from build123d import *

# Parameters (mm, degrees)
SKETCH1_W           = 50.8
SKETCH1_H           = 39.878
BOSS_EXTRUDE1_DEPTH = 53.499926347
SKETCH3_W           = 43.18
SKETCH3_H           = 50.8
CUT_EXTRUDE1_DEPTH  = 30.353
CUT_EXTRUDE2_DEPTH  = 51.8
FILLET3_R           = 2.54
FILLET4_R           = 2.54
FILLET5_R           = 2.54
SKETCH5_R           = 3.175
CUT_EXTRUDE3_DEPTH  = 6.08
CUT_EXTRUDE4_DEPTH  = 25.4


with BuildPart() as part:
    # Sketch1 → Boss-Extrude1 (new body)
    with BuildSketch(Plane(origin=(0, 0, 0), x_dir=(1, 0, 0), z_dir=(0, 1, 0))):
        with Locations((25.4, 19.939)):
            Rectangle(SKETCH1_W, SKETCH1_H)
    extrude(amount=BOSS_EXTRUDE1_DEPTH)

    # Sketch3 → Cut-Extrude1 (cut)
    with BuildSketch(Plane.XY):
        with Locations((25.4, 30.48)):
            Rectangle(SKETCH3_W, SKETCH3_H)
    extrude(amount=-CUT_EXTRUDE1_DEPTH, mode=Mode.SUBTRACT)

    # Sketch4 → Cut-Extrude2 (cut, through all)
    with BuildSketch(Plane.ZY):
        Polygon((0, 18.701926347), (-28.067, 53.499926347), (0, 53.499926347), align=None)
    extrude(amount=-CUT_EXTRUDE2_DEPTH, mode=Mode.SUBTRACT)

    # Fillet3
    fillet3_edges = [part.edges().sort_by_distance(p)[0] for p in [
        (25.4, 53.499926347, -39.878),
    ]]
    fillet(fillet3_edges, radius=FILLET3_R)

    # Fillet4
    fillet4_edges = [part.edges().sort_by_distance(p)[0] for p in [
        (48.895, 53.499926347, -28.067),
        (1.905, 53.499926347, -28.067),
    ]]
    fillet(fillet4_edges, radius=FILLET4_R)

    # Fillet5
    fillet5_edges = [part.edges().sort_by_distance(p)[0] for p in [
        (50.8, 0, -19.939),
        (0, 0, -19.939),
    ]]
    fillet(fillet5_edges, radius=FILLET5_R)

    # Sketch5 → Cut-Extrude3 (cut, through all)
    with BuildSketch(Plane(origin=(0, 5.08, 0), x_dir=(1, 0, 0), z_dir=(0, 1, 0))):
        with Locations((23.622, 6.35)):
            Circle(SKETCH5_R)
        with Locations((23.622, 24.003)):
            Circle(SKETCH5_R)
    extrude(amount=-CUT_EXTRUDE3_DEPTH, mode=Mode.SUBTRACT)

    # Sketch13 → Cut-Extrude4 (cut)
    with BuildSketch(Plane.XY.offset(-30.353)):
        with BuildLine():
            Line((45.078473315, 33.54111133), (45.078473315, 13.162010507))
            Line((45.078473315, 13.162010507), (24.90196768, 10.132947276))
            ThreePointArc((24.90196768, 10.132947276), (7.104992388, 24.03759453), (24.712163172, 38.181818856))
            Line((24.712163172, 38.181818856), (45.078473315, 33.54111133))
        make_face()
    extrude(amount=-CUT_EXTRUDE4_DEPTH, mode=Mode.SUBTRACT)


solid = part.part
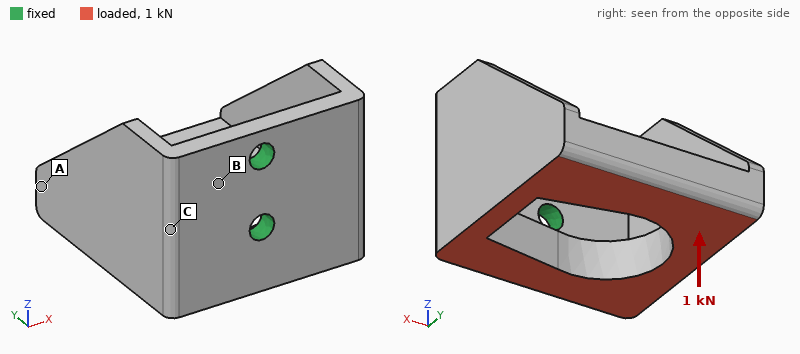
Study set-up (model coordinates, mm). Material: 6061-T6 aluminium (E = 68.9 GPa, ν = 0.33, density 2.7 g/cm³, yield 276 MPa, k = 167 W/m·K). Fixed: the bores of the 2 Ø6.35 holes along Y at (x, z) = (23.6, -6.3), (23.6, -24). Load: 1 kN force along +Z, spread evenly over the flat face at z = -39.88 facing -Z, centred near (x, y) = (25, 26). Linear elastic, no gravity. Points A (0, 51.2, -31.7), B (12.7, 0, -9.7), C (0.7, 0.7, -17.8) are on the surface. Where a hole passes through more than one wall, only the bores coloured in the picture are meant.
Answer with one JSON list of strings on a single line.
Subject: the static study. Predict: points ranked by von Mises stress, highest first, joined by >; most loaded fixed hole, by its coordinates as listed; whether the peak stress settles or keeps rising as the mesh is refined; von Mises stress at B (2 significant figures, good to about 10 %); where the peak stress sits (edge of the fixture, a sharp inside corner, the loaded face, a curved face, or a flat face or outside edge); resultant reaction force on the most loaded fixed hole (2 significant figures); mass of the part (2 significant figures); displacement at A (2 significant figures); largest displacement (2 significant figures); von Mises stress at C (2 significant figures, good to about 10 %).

["B > C > A", "(23.6, -24)", "keeps rising", "31 MPa", "edge of the fixture", "1.1 kN", "86 g", "0.12 mm", "0.15 mm", "16 MPa"]
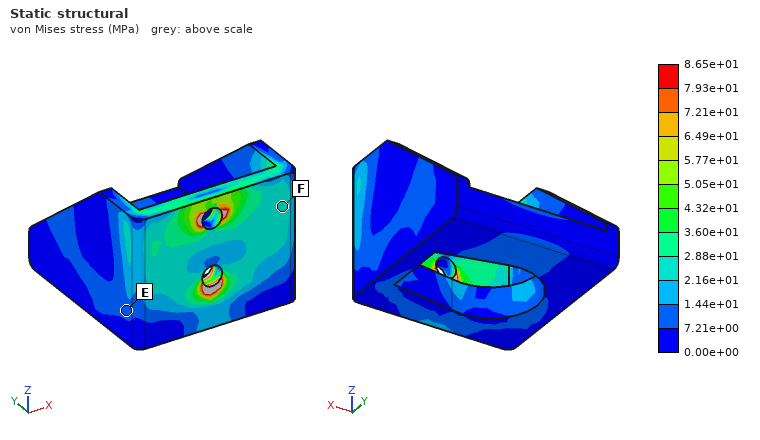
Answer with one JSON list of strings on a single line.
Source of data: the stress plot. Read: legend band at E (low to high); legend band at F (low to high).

["7.21e+00 to 1.44e+01 MPa", "2.16e+01 to 2.88e+01 MPa"]
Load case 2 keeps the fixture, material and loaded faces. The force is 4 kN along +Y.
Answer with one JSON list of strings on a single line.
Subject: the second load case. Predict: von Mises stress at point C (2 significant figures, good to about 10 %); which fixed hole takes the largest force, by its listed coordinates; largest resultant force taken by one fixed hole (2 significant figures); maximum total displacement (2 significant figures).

["32 MPa", "(23.6, -24)", "5.6 kN", "0.37 mm"]
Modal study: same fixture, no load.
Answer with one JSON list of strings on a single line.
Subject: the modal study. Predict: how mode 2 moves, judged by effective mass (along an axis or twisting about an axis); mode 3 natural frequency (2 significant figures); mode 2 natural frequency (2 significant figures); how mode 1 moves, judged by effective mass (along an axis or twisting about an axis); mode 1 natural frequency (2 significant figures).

["along Z", "4000 Hz", "1900 Hz", "along X", "1500 Hz"]
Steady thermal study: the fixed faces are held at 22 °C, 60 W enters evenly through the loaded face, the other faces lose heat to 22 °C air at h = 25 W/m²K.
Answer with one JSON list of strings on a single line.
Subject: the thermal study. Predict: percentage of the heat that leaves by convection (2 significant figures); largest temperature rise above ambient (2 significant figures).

["11 %", "42 K"]
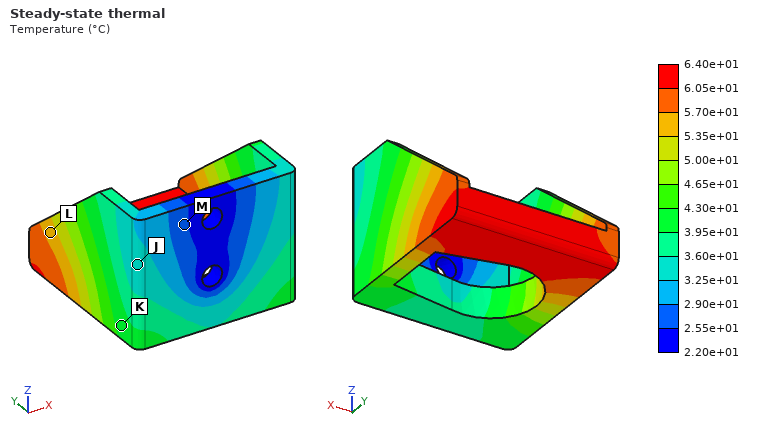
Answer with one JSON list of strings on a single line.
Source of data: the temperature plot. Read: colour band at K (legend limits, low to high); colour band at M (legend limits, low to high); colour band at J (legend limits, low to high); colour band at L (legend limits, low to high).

["3.95e+01 to 4.30e+01 °C", "2.55e+01 to 2.90e+01 °C", "3.25e+01 to 3.60e+01 °C", "5.35e+01 to 5.70e+01 °C"]
